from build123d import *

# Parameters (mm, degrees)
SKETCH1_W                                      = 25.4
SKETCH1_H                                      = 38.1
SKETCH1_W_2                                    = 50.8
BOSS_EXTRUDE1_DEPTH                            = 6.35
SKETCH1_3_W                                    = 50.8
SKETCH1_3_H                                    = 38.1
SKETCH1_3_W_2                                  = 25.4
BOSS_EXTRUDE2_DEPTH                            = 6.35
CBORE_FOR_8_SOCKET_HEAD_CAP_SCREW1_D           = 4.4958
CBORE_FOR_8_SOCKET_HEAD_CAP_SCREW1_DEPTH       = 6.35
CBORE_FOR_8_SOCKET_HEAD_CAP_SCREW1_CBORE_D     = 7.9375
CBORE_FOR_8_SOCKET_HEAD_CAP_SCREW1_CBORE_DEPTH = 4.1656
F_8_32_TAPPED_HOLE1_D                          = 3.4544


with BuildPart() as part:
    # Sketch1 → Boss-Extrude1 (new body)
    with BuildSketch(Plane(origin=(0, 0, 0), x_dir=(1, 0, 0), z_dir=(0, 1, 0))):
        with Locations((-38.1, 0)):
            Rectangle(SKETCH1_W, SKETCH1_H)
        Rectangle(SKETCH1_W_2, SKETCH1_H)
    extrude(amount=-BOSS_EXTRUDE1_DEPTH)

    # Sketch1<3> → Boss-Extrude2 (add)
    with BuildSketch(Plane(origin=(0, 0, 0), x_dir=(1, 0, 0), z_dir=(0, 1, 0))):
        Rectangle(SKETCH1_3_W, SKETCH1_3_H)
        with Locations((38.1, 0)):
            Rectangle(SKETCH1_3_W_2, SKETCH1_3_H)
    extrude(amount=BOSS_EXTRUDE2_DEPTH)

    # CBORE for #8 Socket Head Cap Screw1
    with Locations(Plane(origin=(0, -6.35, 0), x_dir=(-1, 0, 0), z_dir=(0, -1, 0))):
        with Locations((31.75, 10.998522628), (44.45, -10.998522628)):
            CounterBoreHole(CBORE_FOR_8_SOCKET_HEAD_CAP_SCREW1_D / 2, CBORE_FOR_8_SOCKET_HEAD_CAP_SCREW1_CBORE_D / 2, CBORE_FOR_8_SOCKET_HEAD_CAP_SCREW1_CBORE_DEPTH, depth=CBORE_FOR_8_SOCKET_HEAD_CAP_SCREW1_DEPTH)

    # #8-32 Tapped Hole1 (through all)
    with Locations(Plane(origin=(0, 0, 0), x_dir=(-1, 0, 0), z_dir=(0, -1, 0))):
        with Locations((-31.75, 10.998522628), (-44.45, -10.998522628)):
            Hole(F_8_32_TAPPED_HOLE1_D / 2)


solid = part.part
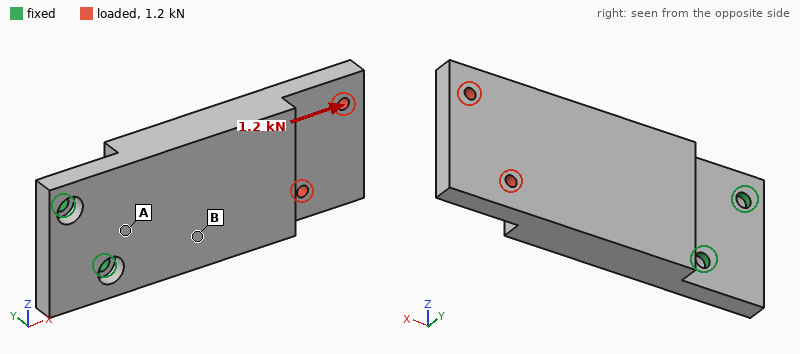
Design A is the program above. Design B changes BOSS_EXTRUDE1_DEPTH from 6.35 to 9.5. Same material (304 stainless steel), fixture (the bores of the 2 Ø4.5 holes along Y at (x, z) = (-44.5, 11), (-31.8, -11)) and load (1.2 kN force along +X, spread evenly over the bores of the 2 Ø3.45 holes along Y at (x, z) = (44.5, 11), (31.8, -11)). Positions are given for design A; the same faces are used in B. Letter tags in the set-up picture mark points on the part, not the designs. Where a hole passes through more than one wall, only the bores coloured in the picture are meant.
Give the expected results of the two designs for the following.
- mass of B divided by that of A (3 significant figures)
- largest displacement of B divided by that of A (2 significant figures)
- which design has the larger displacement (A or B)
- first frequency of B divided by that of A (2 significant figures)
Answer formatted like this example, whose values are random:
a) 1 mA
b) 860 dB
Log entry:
a) 1.24
b) 0.64
c) A
d) 1.2
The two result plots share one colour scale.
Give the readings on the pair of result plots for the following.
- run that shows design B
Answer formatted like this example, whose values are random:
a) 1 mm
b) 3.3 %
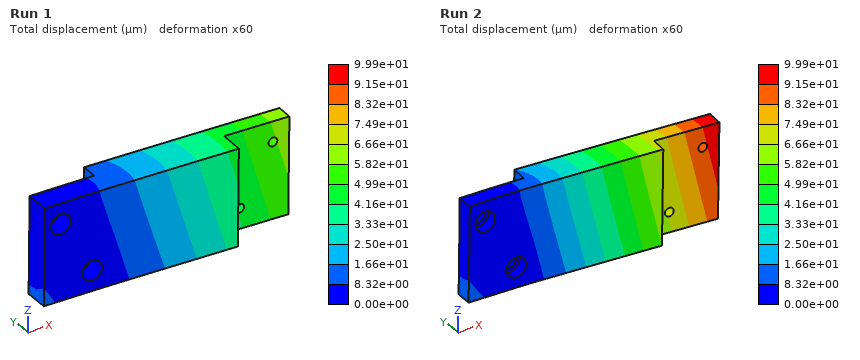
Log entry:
a) Run 1
